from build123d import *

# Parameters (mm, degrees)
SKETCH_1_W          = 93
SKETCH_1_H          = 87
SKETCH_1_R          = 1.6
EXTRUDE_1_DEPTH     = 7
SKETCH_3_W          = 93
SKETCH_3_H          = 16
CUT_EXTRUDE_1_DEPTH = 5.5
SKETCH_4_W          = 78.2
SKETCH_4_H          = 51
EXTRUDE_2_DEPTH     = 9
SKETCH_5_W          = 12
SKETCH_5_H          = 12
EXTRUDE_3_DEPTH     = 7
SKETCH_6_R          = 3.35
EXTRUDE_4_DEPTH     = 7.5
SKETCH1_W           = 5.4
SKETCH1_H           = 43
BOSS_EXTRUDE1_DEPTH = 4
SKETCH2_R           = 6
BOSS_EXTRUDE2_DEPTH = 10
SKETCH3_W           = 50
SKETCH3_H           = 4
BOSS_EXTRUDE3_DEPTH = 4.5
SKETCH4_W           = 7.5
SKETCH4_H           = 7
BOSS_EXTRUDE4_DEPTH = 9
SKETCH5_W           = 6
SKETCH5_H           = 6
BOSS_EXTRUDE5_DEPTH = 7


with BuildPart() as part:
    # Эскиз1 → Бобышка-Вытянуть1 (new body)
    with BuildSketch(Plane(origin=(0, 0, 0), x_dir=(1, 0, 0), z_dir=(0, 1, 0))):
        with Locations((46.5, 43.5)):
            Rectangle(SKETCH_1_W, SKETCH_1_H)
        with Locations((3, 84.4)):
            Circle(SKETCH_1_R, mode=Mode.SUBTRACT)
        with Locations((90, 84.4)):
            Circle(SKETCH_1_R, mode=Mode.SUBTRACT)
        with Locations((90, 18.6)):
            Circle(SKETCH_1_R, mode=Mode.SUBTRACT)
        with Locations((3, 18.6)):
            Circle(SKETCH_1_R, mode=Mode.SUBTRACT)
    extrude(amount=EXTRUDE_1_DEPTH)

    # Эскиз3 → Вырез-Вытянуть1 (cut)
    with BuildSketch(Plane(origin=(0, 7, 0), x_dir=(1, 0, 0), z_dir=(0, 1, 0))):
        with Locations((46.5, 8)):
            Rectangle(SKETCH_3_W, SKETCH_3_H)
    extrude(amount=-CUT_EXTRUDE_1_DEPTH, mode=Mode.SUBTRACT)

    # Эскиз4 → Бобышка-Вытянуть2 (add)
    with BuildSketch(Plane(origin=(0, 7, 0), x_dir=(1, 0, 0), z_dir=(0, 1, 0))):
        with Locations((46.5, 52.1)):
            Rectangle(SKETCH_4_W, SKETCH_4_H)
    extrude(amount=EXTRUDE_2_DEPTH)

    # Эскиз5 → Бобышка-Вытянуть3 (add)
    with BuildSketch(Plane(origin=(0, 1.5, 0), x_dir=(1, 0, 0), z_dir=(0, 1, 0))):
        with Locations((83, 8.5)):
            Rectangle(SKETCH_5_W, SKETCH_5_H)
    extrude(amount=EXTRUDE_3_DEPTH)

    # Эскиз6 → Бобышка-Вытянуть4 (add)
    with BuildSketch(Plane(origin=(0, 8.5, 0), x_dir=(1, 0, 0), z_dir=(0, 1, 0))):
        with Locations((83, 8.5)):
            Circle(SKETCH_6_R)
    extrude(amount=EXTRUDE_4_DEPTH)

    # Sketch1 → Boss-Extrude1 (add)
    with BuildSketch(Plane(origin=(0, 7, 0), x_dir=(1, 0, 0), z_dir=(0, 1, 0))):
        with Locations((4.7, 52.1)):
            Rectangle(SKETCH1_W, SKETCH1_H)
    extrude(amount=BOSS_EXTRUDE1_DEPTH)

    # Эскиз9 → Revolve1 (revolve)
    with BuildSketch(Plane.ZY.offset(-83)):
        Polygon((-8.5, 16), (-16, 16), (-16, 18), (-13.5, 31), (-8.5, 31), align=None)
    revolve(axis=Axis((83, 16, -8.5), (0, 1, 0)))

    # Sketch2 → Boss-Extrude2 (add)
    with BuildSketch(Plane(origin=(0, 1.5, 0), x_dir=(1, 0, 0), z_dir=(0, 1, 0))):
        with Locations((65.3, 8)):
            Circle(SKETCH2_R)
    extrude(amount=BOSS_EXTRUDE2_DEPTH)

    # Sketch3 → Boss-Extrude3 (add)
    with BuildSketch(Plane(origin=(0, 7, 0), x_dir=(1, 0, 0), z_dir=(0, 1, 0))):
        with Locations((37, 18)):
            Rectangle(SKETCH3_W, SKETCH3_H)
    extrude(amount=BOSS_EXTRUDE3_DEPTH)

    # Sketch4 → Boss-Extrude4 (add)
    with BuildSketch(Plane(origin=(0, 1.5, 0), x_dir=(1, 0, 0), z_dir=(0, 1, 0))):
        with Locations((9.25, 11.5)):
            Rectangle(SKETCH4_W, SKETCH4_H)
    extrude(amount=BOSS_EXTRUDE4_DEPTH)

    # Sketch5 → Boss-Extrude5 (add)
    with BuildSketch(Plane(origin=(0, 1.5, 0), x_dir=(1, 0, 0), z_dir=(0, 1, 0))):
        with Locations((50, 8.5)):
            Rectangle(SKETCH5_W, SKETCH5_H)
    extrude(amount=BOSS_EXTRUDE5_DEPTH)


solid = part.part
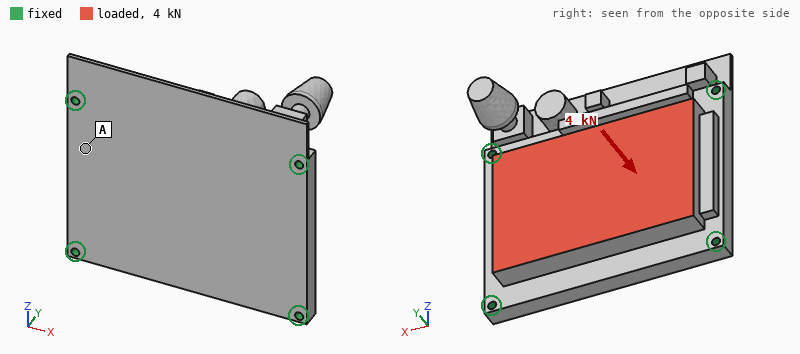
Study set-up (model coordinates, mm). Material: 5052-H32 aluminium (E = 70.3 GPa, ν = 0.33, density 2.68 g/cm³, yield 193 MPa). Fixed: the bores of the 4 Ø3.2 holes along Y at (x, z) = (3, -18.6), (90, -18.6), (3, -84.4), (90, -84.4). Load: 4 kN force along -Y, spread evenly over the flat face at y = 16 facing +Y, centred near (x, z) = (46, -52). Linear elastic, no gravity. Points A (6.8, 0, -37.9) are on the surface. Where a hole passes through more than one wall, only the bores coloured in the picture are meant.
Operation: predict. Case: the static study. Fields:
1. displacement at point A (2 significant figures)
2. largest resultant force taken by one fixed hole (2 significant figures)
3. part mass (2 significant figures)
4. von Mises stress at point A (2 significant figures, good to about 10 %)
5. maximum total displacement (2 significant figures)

16 µm
1.3 kN
240 g
9.2 MPa
31 µm
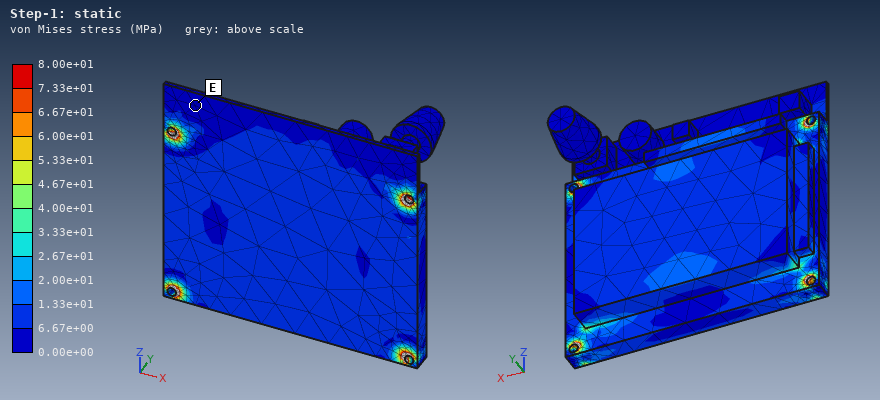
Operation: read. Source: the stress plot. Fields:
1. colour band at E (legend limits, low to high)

0.00e+00 to 6.67e+00 MPa
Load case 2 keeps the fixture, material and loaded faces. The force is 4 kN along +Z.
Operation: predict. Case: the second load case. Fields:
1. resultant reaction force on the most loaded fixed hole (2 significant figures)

1.2 kN
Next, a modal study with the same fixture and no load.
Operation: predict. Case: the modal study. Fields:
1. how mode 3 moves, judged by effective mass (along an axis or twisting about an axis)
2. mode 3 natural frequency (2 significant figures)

along Y
4200 Hz
